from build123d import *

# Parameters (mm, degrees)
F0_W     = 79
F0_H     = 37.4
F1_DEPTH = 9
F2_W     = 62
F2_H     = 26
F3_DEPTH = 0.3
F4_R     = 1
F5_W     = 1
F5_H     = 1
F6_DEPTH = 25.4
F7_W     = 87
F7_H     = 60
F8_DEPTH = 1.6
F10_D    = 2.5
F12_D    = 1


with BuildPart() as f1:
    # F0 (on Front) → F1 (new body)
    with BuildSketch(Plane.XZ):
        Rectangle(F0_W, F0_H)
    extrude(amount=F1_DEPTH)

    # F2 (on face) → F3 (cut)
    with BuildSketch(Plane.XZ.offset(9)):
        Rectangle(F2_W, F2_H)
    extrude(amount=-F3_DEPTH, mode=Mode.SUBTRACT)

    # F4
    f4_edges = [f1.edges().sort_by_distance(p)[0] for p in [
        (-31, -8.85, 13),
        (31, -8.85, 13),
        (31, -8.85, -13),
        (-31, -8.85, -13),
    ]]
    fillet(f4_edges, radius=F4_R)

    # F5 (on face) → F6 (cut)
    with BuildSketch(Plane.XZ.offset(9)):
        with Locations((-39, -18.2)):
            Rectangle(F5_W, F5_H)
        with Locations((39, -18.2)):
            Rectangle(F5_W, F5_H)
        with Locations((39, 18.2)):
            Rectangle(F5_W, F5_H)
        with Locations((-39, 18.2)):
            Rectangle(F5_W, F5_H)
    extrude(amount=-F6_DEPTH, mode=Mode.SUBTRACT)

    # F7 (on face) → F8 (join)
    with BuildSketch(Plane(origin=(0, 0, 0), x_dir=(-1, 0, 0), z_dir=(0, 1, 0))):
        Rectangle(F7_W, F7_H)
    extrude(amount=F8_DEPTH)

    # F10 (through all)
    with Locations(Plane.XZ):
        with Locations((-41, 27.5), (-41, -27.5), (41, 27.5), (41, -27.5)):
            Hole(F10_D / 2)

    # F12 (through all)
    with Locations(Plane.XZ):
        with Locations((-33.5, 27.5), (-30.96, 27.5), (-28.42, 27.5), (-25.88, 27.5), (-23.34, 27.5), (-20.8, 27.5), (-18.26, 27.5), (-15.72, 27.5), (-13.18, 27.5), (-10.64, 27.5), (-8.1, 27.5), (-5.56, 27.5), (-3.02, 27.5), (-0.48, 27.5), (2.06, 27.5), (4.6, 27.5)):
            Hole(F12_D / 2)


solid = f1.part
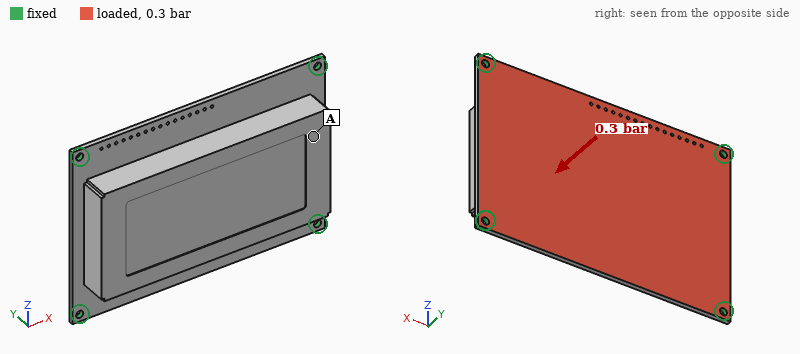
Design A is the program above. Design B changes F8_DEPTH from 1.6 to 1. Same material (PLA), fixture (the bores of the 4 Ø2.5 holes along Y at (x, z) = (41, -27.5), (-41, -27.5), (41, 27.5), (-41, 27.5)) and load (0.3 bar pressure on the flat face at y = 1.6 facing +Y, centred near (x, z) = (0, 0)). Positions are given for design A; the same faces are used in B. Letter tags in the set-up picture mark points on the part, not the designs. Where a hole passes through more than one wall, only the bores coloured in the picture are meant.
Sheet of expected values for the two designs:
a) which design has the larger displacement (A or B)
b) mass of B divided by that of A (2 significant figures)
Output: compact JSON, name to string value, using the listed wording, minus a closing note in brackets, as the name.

{"which design has the larger displacement": "B", "mass of B divided by that of A": "0.91"}
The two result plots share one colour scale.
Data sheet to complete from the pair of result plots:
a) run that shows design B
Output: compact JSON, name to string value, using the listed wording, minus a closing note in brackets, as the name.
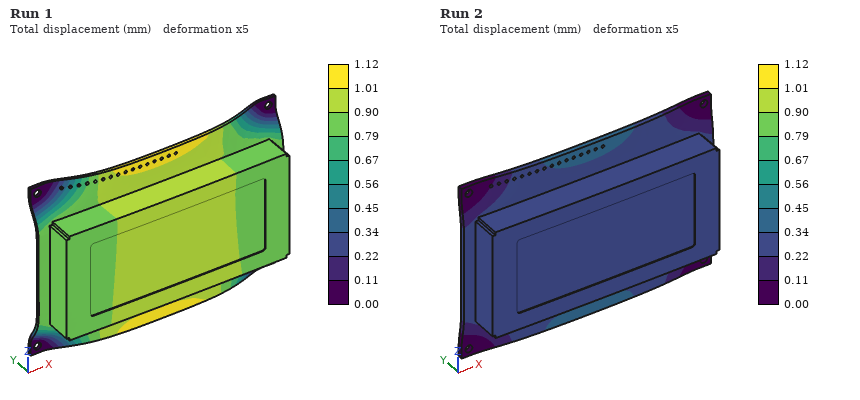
{"run that shows design B": "Run 1"}
